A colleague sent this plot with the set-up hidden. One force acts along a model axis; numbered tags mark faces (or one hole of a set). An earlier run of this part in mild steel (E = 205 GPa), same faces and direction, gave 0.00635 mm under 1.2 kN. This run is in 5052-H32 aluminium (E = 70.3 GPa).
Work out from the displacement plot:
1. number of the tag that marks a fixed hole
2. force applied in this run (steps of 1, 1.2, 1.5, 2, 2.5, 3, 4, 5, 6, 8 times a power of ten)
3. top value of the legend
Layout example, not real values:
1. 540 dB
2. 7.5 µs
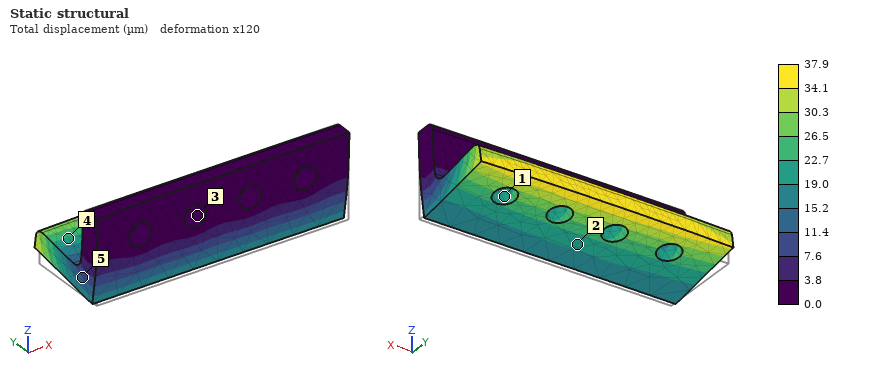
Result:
1. 3
2. 2.5 kN
3. 37.9 µm
